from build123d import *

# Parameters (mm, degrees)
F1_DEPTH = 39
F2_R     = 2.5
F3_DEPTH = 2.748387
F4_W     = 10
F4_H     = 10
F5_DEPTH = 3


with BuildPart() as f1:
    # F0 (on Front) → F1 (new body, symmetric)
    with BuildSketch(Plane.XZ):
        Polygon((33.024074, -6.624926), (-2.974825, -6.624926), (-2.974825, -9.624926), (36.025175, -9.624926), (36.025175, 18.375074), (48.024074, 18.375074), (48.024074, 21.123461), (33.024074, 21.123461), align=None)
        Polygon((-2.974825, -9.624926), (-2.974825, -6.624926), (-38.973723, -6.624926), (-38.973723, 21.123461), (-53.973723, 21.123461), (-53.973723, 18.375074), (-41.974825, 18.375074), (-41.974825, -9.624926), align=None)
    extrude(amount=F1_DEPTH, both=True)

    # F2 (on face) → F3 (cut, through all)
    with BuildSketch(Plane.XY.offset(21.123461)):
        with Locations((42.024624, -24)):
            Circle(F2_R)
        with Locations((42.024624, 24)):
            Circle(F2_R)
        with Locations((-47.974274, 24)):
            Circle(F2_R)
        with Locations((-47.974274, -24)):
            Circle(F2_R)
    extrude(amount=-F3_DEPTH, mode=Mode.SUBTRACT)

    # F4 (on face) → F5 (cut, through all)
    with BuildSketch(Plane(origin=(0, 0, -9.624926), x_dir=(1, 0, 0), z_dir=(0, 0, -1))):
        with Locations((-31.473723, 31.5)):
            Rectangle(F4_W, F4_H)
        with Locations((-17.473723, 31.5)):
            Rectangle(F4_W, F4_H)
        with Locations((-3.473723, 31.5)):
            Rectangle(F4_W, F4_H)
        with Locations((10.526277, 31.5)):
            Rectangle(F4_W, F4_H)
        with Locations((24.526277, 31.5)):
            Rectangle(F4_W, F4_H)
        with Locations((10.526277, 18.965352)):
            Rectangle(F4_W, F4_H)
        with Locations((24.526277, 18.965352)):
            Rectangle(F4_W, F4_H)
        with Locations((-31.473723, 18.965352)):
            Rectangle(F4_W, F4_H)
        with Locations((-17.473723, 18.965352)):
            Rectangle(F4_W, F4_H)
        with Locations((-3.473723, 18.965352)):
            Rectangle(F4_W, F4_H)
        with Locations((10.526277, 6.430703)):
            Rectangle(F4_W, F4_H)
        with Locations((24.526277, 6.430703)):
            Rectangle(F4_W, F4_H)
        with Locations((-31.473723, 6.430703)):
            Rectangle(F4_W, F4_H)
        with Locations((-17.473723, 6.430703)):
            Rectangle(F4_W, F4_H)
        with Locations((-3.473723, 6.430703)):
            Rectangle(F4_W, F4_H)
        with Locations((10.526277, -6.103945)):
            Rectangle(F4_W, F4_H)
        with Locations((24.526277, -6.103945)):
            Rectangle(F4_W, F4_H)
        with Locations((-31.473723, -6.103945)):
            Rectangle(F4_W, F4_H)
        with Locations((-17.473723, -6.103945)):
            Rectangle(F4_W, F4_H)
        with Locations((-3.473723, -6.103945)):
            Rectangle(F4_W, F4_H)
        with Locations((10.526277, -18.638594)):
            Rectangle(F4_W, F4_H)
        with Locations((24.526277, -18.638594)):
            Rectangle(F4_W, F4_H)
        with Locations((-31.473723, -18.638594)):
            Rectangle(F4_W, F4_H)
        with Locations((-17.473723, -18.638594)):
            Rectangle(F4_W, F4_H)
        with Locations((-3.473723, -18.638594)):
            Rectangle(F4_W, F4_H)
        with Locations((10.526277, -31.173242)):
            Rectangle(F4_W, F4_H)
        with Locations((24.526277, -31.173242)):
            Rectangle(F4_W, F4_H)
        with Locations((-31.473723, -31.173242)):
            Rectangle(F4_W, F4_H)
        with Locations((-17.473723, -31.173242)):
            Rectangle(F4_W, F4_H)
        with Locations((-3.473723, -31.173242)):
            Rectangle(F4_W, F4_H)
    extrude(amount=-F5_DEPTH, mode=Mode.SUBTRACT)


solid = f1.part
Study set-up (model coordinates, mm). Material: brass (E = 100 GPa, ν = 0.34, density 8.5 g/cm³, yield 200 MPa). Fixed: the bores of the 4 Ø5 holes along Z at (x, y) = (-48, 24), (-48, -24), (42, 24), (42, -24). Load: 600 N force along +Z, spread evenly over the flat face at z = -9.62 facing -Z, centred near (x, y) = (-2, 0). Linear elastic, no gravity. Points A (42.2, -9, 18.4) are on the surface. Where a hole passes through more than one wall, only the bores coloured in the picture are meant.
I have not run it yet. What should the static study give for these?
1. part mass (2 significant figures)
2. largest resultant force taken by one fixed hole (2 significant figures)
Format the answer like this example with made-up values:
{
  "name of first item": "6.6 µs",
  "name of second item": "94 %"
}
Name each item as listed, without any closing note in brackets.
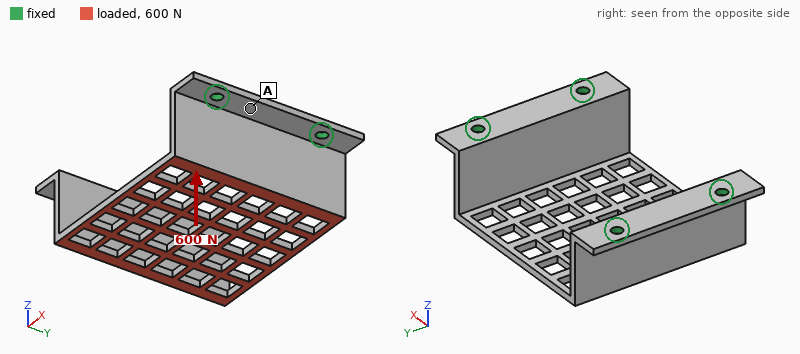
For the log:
{
  "part mass": "230 g",
  "largest resultant force taken by one fixed hole": "170 N"
}
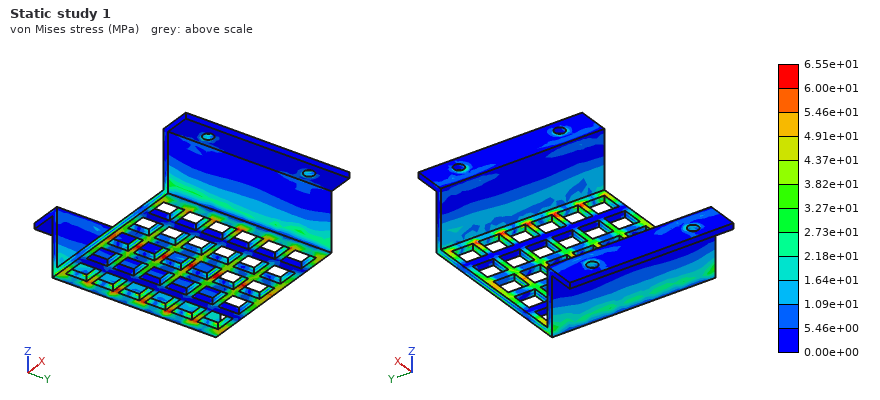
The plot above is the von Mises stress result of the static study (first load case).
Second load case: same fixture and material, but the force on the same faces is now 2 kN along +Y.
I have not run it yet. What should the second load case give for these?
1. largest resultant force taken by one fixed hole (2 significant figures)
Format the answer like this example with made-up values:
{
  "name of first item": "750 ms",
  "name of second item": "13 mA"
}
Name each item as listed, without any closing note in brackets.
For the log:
{
  "largest resultant force taken by one fixed hole": "810 N"
}
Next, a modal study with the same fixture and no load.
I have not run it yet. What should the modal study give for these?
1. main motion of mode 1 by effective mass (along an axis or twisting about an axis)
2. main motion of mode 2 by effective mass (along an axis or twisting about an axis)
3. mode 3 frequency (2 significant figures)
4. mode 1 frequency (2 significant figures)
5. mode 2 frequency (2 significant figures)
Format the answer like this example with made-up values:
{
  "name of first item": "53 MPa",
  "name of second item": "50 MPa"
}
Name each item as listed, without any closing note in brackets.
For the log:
{
  "main motion of mode 1 by effective mass": "along X",
  "main motion of mode 2 by effective mass": "along Z",
  "mode 3 frequency": "1700 Hz",
  "mode 1 frequency": "930 Hz",
  "mode 2 frequency": "1400 Hz"
}
